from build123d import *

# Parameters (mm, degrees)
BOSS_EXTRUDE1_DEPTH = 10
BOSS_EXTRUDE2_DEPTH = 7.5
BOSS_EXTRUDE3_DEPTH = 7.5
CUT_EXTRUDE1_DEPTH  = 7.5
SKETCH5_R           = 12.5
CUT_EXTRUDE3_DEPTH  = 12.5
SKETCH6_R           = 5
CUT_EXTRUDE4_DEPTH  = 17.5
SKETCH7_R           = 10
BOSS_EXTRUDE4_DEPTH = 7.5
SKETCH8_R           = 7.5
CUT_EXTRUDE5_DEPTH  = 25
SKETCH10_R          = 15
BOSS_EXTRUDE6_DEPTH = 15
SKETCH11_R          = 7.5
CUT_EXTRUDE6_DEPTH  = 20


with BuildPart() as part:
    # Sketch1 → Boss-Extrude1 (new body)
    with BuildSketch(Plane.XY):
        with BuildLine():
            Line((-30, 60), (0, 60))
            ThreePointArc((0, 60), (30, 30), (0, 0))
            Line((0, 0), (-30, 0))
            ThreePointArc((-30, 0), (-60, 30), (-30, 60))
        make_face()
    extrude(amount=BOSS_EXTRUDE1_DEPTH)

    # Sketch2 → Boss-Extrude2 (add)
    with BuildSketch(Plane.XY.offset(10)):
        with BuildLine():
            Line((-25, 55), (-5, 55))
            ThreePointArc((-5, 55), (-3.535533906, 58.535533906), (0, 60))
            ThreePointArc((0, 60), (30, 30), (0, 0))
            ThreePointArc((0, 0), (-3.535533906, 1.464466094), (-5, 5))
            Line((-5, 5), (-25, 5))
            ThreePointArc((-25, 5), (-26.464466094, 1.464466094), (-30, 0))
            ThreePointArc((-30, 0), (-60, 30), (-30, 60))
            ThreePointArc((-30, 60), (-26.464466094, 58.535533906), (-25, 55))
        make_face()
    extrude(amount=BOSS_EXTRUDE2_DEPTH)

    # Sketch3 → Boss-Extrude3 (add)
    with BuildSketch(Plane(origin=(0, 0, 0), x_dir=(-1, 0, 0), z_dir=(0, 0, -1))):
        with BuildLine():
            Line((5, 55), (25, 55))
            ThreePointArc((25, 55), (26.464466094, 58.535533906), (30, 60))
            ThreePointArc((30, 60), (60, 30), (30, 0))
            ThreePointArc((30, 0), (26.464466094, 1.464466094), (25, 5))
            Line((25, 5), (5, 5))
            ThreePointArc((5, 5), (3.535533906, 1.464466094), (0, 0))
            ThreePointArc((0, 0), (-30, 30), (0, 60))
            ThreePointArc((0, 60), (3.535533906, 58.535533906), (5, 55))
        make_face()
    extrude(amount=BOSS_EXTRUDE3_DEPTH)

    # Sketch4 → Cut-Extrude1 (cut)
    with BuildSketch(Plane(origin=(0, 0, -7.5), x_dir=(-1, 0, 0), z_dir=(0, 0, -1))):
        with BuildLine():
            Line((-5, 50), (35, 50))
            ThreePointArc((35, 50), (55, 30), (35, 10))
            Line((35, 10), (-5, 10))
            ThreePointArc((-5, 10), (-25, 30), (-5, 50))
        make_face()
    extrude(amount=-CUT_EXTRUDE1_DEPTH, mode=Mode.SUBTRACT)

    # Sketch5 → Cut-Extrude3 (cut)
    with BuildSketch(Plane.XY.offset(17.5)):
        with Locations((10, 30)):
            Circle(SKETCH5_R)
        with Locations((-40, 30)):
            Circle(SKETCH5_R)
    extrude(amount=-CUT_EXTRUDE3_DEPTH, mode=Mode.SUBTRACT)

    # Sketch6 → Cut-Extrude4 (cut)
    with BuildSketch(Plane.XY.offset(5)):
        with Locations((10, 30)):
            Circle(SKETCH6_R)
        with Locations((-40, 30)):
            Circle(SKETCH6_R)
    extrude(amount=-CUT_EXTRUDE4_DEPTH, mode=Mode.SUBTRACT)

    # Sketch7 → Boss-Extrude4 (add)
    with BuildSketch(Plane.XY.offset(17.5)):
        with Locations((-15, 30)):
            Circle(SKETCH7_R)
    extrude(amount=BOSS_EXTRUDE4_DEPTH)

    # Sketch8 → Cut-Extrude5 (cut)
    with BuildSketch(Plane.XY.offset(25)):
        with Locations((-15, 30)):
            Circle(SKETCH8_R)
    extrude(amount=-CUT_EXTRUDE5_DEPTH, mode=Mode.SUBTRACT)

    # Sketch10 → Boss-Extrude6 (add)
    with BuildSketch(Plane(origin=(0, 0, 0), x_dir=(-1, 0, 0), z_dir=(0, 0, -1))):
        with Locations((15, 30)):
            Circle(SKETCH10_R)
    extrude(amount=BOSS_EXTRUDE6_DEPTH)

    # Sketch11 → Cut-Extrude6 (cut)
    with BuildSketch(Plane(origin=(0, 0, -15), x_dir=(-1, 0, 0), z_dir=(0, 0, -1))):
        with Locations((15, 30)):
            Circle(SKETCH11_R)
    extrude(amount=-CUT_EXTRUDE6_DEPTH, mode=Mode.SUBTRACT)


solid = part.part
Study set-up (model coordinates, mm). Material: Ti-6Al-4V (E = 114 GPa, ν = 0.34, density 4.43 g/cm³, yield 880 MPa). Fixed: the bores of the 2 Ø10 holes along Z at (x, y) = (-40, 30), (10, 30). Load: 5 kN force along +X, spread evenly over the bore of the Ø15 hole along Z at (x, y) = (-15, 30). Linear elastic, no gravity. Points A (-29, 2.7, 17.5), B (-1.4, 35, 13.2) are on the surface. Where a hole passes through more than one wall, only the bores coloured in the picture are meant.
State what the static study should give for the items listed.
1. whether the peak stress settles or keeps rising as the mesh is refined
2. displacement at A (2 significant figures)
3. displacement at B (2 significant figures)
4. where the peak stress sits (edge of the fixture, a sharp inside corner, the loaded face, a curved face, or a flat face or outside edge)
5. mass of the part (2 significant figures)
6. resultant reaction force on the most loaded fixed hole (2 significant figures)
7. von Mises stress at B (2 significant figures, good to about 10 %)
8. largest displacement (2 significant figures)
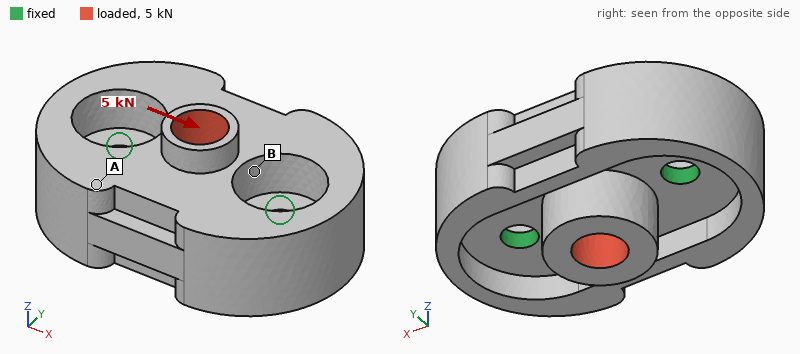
keeps rising
2.1 µm
2.8 µm
edge of the fixture
370 g
2.5 kN
6.1 MPa
5.6 µm
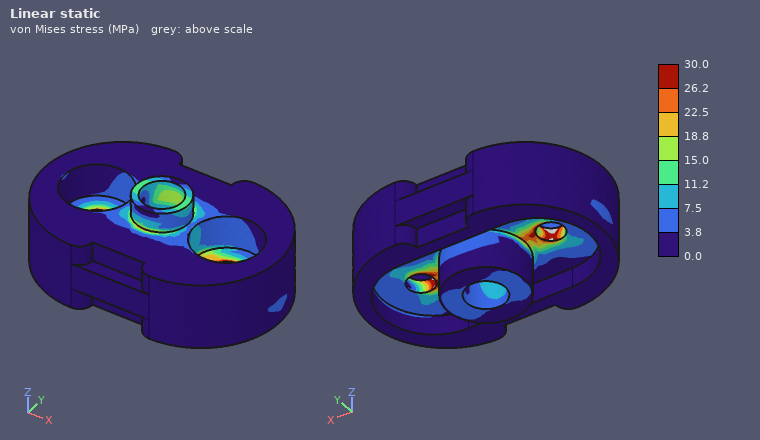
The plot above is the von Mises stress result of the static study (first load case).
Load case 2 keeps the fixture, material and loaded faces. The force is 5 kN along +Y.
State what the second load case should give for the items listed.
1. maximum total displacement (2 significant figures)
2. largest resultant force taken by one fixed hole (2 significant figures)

12 µm
2.5 kN
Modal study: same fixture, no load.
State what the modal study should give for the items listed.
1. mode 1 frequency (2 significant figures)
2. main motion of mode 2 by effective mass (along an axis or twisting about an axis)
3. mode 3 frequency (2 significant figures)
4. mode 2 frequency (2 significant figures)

3200 Hz
along Z
8900 Hz
8000 Hz
